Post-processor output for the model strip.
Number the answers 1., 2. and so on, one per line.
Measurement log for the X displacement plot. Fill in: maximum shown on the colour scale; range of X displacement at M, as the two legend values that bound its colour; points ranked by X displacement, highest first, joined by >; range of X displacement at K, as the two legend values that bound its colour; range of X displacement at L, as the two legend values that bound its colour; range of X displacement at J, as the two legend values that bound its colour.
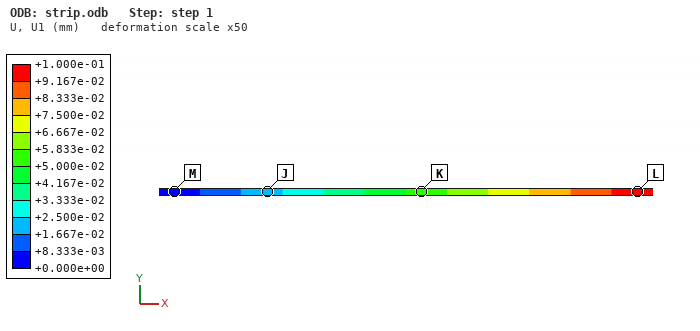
1. +1.000e-01 mm
2. +0.000e+00 to +8.333e-03 mm
3. L > K > J > M
4. +5.000e-02 to +5.833e-02 mm
5. +9.167e-02 to +1.000e-01 mm
6. +1.667e-02 to +2.500e-02 mm
